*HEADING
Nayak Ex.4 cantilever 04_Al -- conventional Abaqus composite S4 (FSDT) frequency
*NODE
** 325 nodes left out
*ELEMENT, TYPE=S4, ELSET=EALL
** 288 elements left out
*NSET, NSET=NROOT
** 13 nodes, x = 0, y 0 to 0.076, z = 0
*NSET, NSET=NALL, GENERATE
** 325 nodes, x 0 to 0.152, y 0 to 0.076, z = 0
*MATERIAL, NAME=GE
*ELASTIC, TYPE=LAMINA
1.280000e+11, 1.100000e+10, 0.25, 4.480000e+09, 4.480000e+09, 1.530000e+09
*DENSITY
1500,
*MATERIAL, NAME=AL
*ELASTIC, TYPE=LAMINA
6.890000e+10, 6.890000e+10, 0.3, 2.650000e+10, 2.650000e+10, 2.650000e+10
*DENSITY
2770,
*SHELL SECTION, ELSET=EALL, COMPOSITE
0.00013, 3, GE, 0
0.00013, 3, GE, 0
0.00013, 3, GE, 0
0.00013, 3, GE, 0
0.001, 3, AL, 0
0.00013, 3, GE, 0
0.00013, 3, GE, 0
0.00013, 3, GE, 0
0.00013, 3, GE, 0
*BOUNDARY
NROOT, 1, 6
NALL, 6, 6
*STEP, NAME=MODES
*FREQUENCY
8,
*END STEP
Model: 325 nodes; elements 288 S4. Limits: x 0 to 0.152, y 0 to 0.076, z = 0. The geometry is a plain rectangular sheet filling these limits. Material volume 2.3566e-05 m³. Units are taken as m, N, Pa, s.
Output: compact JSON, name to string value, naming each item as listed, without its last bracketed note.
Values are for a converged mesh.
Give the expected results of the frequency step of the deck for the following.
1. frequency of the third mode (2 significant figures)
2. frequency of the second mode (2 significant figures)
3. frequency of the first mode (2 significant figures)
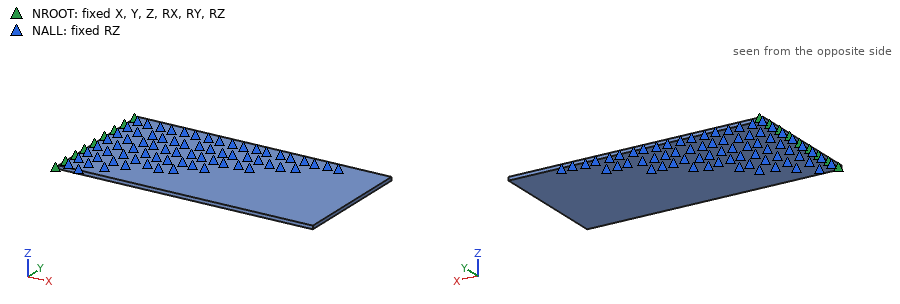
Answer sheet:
{"frequency of the third mode": "680 Hz", "frequency of the second mode": "230 Hz", "frequency of the first mode": "110 Hz"}
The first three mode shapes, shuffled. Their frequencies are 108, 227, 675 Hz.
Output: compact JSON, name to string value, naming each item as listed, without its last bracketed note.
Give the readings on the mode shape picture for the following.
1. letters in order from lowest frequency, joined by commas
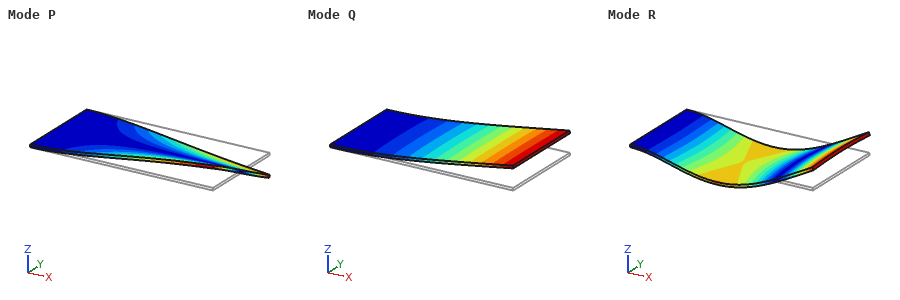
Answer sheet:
{"letters in order from lowest frequency, joined by commas": "Q, P, R"}
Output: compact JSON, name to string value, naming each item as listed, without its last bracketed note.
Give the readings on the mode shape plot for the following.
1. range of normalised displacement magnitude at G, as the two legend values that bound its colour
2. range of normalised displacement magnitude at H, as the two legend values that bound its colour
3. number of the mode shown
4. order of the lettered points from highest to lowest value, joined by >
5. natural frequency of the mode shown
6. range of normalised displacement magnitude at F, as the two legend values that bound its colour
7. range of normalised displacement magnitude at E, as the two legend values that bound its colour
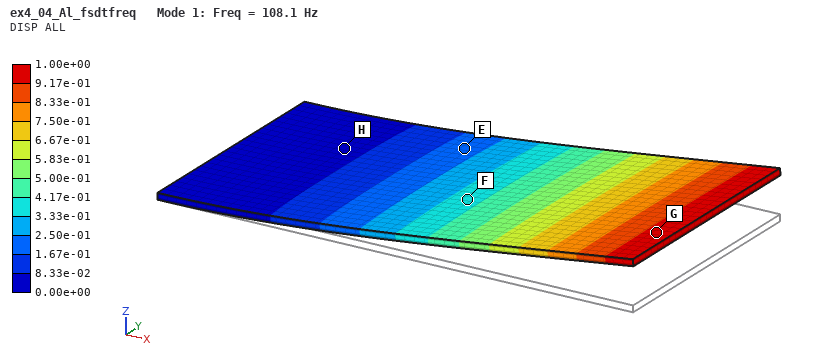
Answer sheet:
{"range of normalised displacement magnitude at G, as the two legend values that bound its colour": "9.17e-01 to 1.00e+00", "range of normalised displacement magnitude at H, as the two legend values that bound its colour": "0.00e+00 to 8.33e-02", "number of the mode shown": "1", "order of the lettered points from highest to lowest value, joined by >": "G > F > E > H", "natural frequency of the mode shown": "108.1 Hz", "range of normalised displacement magnitude at F, as the two legend values that bound its colour": "3.33e-01 to 4.17e-01", "range of normalised displacement magnitude at E, as the two legend values that bound its colour": "1.67e-01 to 2.50e-01"}
